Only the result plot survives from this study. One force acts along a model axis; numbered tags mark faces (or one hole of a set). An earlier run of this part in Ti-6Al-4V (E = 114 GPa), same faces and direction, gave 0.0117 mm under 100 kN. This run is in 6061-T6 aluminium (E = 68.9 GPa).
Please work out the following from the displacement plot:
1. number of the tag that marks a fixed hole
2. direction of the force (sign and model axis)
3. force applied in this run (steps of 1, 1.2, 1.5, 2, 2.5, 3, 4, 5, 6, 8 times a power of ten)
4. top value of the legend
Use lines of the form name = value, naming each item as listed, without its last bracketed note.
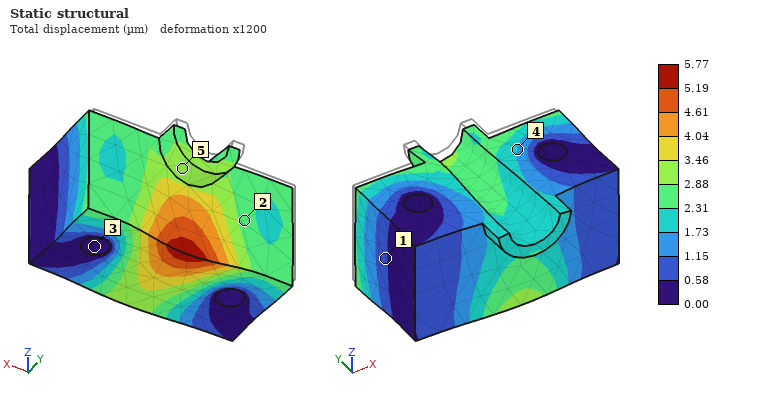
number of the tag that marks a fixed hole = 3
direction of the force = -Y
force applied in this run = 30 kN
top value of the legend = 5.77 µm
